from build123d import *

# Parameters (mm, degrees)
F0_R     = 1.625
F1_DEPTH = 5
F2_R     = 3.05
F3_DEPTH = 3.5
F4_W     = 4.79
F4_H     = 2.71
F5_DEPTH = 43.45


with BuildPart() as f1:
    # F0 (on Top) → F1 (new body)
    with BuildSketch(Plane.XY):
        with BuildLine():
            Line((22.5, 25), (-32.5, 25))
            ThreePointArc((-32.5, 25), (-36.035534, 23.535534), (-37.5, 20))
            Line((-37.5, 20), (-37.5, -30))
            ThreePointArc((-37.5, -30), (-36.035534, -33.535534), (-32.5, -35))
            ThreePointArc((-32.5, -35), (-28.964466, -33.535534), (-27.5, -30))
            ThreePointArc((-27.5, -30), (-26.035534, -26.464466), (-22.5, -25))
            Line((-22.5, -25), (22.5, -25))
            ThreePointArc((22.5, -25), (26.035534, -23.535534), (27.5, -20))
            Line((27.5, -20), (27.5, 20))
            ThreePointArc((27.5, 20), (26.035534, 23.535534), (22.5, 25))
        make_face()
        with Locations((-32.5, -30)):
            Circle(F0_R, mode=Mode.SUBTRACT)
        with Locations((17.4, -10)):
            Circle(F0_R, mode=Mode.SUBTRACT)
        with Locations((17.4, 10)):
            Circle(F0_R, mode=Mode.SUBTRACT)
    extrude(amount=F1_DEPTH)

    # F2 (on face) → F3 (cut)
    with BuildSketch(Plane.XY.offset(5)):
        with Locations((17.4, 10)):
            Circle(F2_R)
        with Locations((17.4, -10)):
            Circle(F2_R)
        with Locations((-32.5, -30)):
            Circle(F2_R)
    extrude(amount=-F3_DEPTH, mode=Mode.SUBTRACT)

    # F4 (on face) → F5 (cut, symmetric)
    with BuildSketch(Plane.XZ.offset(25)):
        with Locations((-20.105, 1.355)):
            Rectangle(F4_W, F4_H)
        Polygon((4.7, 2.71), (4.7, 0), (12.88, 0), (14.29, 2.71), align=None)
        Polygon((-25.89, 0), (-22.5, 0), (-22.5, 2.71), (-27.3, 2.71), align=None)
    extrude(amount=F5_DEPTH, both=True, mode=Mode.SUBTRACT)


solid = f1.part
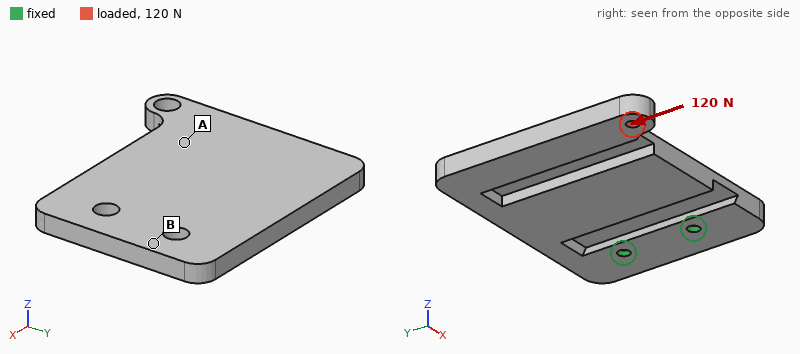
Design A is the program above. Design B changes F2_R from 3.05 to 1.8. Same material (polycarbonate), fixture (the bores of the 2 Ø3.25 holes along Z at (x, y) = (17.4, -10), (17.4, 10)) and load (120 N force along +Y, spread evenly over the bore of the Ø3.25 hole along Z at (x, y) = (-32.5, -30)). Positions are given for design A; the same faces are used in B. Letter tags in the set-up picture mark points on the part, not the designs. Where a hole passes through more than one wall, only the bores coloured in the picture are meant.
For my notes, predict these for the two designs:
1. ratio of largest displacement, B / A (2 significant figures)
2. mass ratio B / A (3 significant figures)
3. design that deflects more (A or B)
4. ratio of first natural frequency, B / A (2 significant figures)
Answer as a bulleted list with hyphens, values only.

- 0.86
- 1.01
- A
- 1.1
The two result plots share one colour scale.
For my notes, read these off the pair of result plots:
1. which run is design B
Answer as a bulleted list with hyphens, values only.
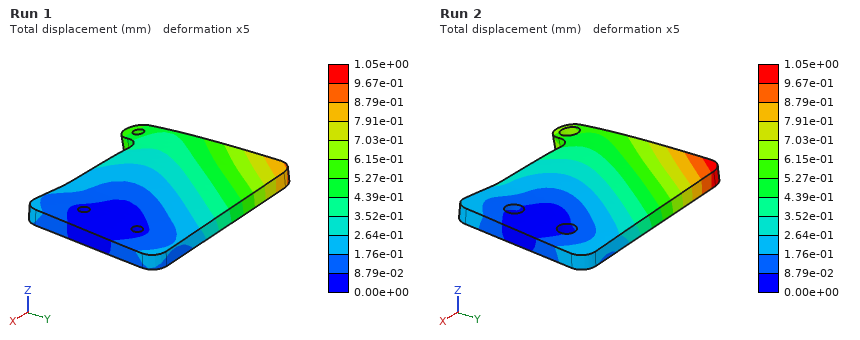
- Run 1
